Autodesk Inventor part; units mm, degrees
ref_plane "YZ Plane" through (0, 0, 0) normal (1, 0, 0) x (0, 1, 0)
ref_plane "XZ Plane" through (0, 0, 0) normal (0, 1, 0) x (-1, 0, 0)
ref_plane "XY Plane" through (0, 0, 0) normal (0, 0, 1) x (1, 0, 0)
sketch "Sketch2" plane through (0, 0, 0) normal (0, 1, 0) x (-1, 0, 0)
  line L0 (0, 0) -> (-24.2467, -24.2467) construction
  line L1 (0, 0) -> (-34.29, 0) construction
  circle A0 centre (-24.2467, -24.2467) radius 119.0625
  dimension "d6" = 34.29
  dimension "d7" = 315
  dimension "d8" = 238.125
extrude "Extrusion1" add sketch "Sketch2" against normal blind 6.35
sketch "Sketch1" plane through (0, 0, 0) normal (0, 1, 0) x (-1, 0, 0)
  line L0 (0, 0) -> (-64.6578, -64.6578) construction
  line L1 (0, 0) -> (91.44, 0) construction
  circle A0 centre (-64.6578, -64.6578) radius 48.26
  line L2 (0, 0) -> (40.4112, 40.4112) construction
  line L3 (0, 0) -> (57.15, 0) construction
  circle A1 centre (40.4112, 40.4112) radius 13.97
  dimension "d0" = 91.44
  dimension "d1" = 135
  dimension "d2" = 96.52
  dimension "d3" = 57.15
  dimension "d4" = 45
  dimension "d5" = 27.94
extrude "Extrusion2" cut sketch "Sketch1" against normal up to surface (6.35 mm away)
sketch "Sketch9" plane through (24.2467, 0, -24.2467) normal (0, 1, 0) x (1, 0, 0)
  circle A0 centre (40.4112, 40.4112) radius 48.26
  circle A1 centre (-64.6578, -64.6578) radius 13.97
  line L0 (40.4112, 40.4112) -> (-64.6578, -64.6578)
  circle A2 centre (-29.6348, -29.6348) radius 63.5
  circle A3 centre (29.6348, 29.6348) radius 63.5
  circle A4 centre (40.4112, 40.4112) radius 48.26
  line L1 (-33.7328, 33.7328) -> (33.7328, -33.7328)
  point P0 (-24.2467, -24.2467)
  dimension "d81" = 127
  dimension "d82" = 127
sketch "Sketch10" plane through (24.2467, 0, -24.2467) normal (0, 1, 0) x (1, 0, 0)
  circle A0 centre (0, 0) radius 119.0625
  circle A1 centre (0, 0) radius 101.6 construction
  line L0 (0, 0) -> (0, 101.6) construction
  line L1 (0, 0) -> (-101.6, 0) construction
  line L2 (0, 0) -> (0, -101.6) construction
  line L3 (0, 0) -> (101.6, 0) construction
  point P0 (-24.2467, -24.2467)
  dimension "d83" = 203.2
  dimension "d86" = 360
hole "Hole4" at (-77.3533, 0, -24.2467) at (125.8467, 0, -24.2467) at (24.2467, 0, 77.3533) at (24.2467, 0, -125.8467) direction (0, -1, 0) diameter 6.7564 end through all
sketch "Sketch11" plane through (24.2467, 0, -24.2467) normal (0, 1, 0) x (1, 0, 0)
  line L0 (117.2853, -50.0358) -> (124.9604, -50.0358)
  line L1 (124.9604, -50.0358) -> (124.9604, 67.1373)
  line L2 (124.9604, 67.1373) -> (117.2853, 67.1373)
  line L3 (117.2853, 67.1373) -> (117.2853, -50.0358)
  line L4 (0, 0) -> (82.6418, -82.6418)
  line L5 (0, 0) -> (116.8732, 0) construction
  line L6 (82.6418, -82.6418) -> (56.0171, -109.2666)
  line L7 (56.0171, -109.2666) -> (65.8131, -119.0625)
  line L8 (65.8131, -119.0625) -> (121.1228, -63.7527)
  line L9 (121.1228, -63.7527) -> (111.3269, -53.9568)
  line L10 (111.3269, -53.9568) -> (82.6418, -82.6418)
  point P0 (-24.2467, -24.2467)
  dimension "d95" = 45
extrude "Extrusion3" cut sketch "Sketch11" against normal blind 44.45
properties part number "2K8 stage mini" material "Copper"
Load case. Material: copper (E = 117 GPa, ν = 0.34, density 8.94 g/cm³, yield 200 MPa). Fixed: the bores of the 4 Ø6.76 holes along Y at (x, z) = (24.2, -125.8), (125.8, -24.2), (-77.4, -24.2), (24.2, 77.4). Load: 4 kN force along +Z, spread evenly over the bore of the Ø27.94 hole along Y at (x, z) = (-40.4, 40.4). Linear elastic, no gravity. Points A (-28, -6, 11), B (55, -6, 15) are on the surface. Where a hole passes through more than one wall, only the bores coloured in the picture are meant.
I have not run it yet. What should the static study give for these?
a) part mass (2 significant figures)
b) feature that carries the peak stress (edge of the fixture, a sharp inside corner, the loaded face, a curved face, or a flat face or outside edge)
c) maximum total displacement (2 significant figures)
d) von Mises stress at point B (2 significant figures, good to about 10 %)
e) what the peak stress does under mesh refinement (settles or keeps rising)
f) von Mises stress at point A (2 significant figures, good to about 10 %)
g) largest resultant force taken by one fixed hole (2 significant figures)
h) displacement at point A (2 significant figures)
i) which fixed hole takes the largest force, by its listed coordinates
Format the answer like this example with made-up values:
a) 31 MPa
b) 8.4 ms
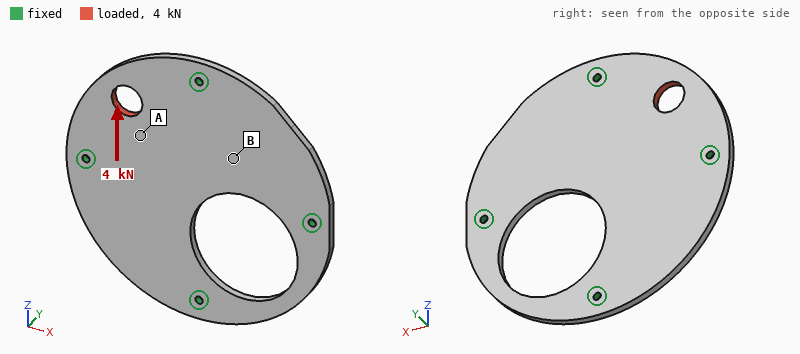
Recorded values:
a) 2.1 kg
b) edge of the fixture
c) 8.4 µm
d) 2.0 MPa
e) keeps rising
f) 5.7 MPa
g) 2.0 kN
h) 4.2 µm
i) (-77.4, -24.2)
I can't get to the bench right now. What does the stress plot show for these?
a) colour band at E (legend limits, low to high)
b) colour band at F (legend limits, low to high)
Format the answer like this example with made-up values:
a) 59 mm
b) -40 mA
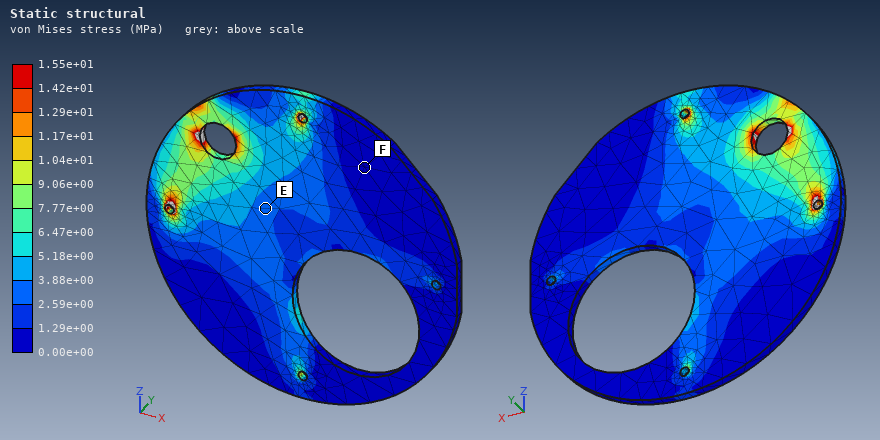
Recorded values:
a) 2.59e+00 to 3.88e+00 MPa
b) 0.00e+00 to 1.29e+00 MPa
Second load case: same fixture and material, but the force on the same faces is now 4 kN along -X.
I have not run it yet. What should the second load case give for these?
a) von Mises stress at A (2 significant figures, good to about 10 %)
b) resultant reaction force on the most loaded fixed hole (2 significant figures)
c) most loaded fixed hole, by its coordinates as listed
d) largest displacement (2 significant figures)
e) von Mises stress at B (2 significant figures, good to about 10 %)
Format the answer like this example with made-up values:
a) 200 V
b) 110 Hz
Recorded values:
a) 5.6 MPa
b) 2.0 kN
c) (24.2, 77.4)
d) 8.5 µm
e) 2.9 MPa
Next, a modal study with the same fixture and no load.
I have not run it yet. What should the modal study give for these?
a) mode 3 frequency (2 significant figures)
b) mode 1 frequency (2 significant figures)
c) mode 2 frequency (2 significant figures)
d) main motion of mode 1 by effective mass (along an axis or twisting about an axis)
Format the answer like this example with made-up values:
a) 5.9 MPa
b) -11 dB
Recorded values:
a) 900 Hz
b) 770 Hz
c) 860 Hz
d) along Y
